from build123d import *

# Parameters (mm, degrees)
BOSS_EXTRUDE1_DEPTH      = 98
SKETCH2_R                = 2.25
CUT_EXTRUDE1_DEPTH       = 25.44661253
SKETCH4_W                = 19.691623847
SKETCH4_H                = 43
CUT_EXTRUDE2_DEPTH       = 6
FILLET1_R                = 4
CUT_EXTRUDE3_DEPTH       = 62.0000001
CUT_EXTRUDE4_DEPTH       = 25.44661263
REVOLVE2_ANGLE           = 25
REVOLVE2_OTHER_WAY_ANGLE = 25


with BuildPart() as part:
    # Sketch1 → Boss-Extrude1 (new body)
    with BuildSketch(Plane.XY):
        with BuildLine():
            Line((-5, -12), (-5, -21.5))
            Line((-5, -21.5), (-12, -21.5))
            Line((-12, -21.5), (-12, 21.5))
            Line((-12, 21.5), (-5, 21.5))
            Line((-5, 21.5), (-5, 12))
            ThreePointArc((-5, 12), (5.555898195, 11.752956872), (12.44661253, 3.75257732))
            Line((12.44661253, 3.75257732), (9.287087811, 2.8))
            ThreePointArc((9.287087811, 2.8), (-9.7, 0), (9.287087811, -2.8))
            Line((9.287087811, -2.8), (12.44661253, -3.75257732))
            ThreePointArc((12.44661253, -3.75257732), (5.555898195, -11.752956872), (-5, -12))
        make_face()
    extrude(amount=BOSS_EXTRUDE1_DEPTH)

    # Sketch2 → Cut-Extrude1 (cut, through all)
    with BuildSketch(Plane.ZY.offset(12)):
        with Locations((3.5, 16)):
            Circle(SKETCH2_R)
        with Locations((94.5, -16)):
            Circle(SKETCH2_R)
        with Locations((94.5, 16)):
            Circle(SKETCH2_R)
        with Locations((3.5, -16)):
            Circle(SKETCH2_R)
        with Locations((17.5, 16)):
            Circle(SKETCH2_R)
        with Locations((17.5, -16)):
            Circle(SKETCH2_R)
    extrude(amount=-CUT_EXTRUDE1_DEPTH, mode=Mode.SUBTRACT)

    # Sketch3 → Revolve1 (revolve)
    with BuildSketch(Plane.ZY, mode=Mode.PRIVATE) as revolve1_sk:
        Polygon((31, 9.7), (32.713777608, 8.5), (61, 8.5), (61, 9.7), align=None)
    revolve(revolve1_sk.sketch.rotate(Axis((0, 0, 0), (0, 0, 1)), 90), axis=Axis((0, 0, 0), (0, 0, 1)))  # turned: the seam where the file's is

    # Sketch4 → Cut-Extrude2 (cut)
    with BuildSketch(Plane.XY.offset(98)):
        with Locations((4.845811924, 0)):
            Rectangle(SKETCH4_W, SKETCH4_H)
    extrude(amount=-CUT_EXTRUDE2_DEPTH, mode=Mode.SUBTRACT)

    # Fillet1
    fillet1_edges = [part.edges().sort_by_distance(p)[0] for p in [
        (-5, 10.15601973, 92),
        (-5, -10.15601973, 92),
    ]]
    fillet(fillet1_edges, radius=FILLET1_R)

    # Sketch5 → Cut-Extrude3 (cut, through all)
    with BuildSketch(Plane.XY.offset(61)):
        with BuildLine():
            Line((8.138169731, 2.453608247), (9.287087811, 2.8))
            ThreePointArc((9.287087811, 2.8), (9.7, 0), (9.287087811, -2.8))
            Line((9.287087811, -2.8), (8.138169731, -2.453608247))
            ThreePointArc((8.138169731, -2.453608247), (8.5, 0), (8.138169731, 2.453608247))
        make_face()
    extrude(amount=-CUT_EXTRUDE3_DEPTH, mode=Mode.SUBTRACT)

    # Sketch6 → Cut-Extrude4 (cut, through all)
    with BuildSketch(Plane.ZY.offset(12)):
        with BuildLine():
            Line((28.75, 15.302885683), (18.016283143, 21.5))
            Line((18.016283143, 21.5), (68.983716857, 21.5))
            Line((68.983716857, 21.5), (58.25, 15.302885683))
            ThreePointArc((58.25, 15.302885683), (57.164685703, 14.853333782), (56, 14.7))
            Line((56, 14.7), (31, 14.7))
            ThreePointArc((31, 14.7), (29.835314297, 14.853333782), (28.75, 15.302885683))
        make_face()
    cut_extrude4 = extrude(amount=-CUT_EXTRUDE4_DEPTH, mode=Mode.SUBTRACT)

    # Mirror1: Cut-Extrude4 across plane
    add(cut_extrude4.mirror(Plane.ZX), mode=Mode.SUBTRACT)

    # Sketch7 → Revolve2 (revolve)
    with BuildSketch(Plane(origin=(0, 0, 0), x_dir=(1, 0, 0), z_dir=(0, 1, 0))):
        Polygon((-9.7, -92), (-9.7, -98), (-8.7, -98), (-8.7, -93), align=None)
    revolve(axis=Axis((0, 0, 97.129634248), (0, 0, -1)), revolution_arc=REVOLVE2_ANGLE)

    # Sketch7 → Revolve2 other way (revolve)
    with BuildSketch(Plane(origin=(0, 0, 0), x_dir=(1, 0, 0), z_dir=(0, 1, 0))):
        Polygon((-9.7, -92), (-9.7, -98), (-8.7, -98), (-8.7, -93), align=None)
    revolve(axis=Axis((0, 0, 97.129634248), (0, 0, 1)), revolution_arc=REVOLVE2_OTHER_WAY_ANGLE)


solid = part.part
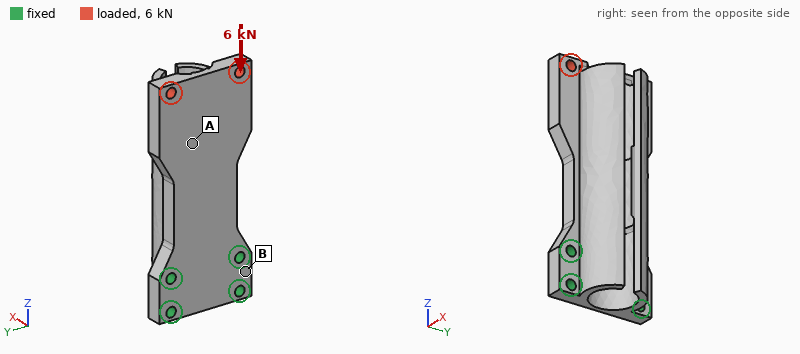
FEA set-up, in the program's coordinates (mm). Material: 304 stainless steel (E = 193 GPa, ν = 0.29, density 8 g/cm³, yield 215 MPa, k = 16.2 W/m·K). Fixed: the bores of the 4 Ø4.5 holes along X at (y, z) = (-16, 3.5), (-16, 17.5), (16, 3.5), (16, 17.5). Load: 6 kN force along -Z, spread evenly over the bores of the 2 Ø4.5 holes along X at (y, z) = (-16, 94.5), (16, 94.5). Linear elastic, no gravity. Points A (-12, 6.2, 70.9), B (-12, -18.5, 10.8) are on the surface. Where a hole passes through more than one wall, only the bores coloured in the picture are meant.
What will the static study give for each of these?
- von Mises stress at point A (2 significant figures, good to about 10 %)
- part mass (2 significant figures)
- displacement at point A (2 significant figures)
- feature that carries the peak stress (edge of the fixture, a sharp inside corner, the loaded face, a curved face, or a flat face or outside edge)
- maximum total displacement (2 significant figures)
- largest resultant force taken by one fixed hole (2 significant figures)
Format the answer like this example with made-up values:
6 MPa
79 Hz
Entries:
29 MPa
270 g
17 µm
the loaded face
34 µm
2.4 kN
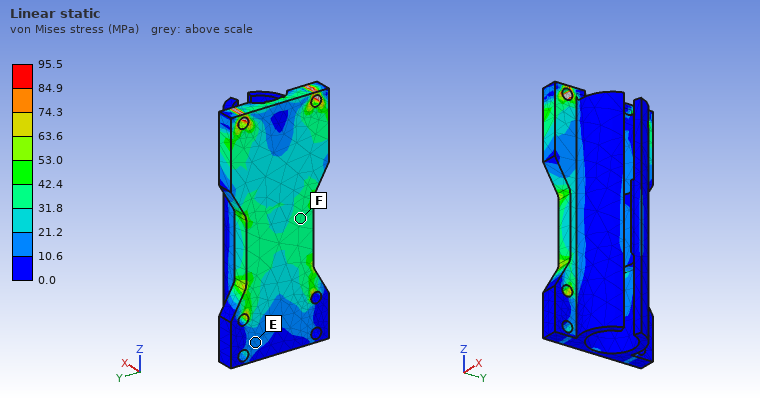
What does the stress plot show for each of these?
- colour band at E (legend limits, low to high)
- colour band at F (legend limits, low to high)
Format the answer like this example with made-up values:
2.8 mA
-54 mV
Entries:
10.6 to 21.2 MPa
31.8 to 42.4 MPa
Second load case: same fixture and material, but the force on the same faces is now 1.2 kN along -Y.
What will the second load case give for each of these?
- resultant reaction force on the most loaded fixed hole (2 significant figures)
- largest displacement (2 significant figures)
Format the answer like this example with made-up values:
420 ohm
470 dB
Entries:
2.7 kN
67 µm
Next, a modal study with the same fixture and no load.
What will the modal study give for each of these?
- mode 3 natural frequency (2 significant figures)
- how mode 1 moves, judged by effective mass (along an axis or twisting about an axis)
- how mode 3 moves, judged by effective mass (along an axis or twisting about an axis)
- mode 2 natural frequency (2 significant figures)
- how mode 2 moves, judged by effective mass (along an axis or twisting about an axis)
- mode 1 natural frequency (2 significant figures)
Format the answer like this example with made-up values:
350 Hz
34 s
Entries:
3500 Hz
along X
along Y
2200 Hz
along Y
1700 Hz
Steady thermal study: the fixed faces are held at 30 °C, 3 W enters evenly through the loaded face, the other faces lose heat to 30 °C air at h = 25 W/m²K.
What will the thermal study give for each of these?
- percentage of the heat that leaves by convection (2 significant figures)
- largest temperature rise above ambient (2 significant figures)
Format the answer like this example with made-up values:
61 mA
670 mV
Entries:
82 %
24 K
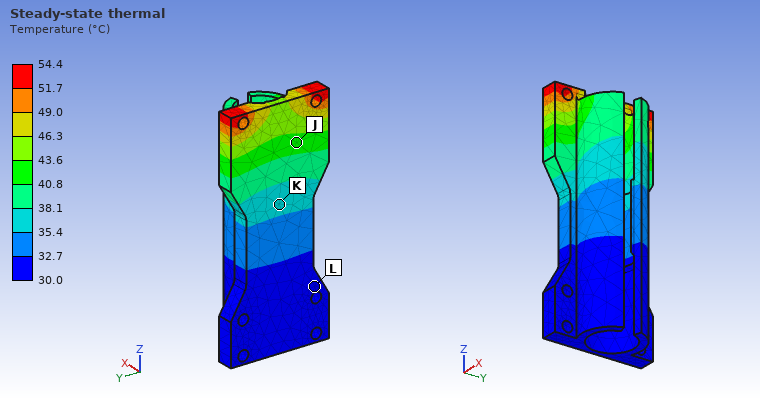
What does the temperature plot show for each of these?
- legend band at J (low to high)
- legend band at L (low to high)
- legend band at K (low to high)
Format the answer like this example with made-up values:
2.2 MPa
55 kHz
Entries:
40.8 to 43.6 °C
30.0 to 32.7 °C
35.4 to 38.1 °C
